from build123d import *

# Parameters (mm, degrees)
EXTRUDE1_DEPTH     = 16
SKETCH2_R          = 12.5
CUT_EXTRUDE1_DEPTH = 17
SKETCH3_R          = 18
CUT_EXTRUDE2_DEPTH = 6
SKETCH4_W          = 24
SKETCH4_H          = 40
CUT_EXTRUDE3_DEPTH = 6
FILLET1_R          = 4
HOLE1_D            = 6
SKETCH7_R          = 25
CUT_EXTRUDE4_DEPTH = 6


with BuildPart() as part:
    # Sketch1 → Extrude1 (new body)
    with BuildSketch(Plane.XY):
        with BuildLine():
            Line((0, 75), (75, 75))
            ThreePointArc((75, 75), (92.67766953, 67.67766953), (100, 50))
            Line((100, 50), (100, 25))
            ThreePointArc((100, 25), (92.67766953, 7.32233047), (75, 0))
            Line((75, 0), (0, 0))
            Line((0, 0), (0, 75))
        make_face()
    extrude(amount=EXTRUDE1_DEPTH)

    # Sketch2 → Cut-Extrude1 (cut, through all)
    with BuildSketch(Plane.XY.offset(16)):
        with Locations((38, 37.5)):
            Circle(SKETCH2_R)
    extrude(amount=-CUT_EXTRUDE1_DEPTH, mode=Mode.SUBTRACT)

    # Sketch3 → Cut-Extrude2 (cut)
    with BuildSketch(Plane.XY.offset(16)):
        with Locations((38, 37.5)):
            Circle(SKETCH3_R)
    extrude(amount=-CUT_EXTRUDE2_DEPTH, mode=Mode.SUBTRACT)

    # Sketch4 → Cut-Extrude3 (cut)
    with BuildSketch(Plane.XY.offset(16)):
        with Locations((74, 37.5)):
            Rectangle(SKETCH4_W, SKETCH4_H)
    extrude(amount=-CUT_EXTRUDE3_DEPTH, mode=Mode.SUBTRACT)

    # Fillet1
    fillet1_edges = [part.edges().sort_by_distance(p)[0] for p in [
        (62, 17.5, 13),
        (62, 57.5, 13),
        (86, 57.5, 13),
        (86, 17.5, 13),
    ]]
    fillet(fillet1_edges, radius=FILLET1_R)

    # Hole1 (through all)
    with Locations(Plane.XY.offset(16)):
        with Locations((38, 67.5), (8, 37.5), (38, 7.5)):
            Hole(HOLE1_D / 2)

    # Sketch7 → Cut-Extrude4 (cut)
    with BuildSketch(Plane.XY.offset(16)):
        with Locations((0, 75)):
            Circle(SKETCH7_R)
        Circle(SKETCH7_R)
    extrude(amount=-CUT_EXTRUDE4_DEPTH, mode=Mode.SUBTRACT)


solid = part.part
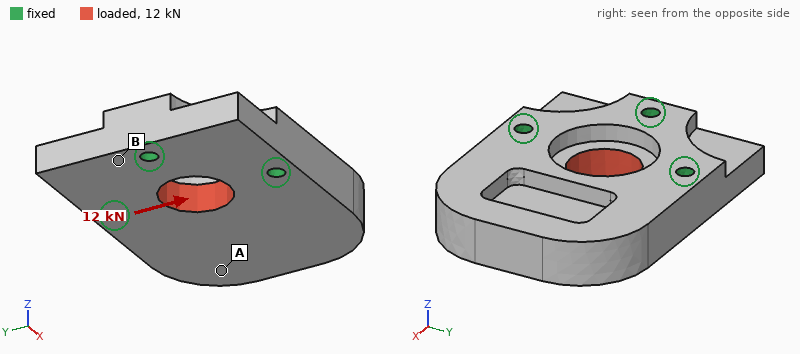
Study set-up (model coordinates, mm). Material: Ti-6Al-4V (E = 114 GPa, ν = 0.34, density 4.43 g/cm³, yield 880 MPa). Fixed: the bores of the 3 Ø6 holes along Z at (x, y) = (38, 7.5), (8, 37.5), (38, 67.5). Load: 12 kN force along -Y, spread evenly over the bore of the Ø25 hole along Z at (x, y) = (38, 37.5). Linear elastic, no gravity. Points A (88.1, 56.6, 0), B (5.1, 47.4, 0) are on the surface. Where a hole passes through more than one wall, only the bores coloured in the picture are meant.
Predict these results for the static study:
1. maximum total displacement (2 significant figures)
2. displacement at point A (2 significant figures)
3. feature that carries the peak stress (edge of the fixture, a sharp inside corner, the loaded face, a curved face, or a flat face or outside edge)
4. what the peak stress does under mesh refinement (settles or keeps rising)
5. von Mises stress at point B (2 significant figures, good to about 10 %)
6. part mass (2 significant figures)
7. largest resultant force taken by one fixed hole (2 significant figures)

5.2 µm
3.4 µm
edge of the fixture
keeps rising
6.5 MPa
410 g
4.9 kN
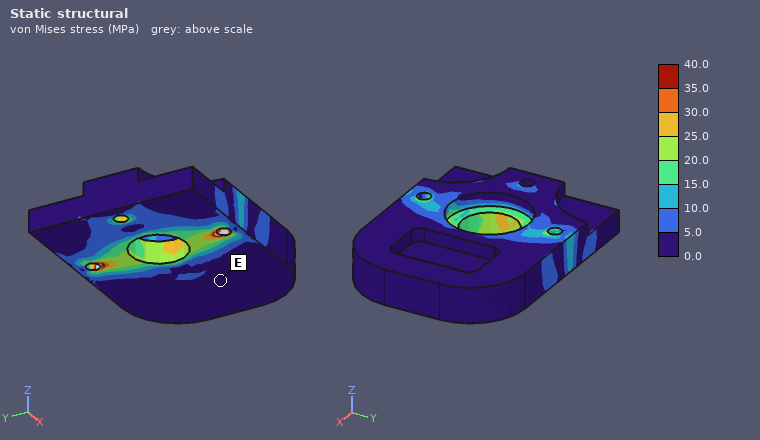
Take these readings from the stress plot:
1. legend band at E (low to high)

0.0 to 5.0 MPa
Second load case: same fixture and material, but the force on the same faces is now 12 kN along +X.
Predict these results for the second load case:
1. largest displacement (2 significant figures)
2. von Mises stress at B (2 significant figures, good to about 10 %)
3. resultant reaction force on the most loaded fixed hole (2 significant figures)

11 µm
8.2 MPa
4.1 kN
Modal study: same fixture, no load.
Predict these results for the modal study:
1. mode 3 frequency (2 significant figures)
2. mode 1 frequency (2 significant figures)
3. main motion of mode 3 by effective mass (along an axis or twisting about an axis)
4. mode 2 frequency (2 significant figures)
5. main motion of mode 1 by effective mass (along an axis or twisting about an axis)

8900 Hz
2900 Hz
along Y
6200 Hz
along Z
